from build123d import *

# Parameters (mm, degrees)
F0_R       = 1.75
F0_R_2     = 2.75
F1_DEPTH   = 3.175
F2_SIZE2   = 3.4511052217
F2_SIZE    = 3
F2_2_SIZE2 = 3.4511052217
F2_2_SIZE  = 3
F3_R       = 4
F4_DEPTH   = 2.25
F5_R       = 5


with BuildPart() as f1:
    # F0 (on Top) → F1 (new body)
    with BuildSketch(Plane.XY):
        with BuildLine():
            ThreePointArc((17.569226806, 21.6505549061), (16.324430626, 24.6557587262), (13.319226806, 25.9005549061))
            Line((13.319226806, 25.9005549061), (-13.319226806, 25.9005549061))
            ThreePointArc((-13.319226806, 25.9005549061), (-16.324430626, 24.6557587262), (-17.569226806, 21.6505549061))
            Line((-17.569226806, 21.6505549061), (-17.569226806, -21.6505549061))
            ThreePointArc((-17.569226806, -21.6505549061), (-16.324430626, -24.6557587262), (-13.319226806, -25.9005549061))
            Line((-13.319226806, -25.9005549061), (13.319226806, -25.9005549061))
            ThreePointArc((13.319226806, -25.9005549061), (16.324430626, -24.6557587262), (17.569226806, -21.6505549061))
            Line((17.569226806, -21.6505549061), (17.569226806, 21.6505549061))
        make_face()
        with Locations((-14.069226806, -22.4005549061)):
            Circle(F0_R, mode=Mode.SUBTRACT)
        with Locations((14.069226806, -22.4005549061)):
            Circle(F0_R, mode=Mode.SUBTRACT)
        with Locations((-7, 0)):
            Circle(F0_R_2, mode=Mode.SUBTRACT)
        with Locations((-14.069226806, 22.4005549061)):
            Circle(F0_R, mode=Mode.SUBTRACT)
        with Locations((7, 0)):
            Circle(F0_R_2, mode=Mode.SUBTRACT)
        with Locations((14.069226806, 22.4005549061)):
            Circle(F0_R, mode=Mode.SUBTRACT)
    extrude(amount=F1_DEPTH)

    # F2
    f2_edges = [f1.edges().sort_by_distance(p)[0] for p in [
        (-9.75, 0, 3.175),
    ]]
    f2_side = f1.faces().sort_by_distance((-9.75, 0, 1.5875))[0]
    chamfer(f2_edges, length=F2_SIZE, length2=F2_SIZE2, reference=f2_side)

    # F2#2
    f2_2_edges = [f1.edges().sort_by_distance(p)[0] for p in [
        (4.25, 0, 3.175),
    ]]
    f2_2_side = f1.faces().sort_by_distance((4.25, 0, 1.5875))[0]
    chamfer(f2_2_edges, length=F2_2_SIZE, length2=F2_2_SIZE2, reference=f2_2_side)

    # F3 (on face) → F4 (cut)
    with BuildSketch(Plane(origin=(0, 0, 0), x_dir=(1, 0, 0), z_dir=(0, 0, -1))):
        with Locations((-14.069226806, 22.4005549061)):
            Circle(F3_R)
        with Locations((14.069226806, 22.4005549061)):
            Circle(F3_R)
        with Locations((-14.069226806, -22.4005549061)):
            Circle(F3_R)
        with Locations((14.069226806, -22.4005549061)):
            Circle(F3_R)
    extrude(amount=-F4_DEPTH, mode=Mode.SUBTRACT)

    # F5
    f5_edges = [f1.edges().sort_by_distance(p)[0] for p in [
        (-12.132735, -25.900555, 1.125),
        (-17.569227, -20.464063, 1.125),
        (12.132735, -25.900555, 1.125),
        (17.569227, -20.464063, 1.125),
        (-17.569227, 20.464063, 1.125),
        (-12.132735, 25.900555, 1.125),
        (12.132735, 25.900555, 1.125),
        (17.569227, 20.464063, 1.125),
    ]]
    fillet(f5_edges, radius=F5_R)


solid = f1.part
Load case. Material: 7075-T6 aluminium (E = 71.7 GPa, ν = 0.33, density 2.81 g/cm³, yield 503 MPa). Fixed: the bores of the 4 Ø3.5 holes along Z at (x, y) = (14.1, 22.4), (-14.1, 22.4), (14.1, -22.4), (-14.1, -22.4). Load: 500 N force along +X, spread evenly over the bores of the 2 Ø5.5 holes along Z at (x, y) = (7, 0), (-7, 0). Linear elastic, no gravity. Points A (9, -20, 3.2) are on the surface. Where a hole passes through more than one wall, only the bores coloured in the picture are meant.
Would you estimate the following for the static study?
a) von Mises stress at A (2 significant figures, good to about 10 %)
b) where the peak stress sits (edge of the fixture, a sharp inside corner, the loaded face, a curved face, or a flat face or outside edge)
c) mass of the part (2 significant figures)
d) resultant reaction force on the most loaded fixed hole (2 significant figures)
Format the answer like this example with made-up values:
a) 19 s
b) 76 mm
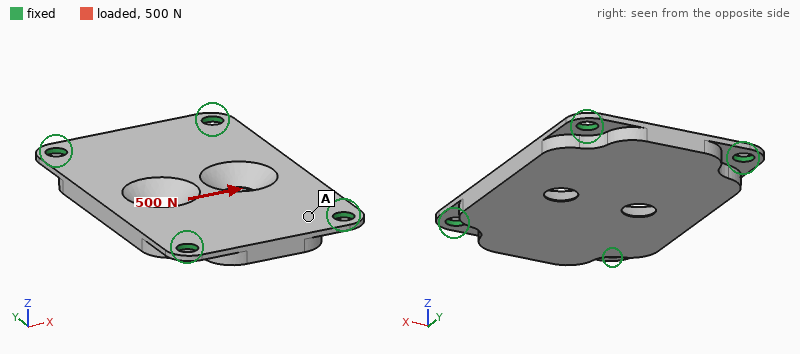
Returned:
a) 9.8 MPa
b) the loaded face
c) 13 g
d) 150 N
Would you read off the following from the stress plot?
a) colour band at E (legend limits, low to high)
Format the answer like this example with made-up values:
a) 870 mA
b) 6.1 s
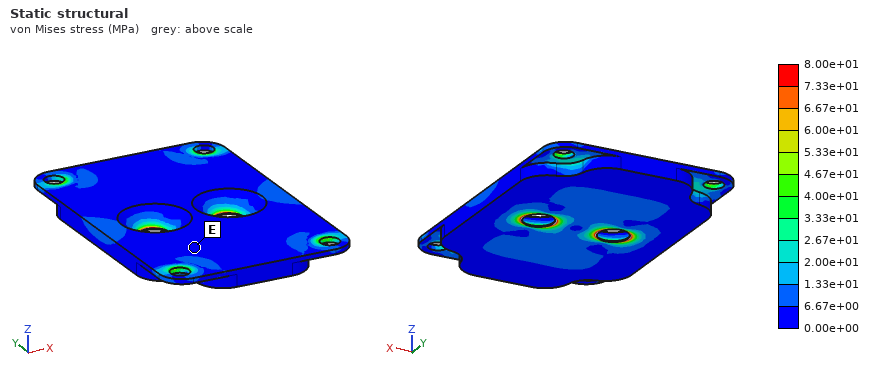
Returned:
a) 0.00e+00 to 6.67e+00 MPa
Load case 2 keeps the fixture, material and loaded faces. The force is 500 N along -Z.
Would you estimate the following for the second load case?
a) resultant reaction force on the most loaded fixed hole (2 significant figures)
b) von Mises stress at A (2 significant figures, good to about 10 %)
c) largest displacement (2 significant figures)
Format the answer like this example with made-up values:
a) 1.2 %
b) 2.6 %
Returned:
a) 540 N
b) 31 MPa
c) 0.12 mm
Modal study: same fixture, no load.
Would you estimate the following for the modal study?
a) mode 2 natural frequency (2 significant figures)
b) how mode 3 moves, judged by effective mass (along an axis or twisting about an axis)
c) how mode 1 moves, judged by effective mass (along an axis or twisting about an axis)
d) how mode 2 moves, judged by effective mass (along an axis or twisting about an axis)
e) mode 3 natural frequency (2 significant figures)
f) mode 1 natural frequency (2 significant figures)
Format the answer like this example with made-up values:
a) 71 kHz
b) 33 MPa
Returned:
a) 8100 Hz
b) twisting about X
c) along Z
d) twisting about Y
e) 12 kHz
f) 5000 Hz
